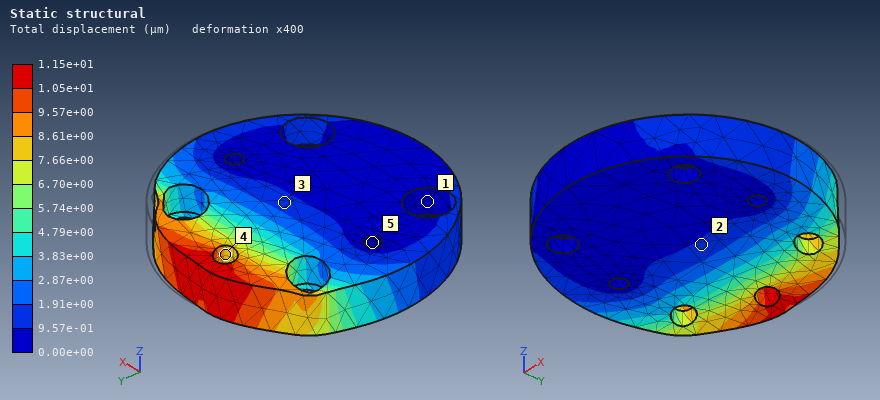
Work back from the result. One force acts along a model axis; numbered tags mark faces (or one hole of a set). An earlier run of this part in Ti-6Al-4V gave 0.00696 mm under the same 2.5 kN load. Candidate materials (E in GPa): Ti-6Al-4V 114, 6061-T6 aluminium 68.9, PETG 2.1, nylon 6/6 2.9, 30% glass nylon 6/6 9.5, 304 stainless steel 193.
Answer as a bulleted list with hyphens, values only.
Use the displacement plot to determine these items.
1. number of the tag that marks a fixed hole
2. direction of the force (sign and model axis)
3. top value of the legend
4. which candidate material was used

- 5
- -X
- 1.15e+01 µm
- 6061-T6 aluminium
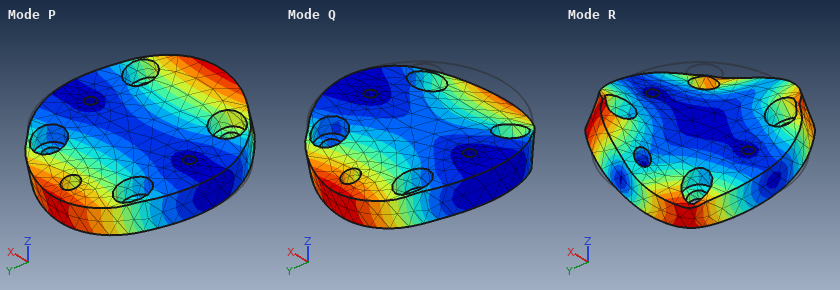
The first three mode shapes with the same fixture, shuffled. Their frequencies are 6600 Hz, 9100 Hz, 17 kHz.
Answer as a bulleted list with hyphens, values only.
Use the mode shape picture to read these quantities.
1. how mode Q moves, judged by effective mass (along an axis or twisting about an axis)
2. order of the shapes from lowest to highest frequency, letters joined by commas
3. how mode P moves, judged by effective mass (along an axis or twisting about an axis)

- along Z
- P, Q, R
- twisting about X
